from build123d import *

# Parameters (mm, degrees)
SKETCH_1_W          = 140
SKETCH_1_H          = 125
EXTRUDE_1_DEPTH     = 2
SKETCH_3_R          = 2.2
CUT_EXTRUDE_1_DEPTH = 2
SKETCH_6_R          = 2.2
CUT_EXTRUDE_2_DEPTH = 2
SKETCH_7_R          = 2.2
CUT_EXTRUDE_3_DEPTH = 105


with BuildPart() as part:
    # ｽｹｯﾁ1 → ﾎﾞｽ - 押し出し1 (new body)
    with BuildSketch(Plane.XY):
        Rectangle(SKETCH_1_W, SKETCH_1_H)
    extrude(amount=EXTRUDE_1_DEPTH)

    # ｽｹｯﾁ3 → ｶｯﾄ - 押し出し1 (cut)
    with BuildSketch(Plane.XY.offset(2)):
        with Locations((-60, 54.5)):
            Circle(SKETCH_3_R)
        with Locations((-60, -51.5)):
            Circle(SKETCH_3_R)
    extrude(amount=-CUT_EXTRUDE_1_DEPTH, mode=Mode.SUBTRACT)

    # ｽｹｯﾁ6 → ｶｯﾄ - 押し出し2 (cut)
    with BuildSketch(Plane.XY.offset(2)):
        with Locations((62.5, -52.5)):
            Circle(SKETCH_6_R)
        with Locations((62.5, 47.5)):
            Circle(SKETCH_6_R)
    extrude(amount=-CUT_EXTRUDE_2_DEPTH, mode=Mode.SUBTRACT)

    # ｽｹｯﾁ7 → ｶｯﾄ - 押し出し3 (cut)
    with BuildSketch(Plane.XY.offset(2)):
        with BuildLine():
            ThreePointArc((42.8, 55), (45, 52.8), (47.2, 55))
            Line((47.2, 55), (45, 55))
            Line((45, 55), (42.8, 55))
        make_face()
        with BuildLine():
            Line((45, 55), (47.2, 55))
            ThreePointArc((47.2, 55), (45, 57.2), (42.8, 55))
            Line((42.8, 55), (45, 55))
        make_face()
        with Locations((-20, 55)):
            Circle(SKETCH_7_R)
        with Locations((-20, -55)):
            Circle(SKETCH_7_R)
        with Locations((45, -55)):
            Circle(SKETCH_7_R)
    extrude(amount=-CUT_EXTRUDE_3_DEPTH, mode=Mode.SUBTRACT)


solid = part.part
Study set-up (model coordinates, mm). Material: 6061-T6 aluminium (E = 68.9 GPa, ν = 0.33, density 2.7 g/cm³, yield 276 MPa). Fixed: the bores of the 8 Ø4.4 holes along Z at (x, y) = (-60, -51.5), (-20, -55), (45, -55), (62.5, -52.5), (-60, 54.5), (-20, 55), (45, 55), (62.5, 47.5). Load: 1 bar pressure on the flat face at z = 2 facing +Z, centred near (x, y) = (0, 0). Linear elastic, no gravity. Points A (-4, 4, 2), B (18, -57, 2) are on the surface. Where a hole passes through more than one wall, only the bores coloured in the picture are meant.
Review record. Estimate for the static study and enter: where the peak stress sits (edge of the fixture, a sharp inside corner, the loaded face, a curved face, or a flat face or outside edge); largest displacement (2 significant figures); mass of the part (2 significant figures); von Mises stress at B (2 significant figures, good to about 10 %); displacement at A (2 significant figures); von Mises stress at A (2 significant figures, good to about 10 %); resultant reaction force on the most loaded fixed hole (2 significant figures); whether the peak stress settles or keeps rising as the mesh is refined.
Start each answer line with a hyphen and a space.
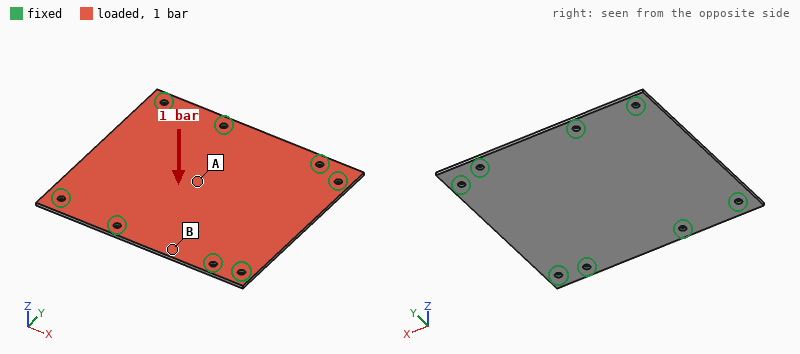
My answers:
- edge of the fixture
- 0.99 mm
- 94 g
- 34 MPa
- 0.97 mm
- 71 MPa
- 330 N
- keeps rising
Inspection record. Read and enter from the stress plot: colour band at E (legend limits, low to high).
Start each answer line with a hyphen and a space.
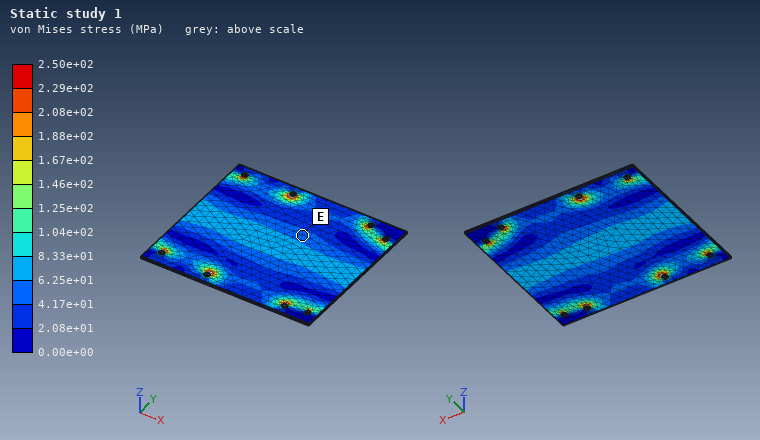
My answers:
- 4.17e+01 to 6.25e+01 MPa
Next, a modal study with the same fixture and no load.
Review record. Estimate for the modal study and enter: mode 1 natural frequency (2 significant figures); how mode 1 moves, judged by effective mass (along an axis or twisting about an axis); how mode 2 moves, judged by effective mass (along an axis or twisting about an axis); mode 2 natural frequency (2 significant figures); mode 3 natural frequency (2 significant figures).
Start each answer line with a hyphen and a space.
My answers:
- 830 Hz
- along Z
- twisting about Y
- 1100 Hz
- 1400 Hz
